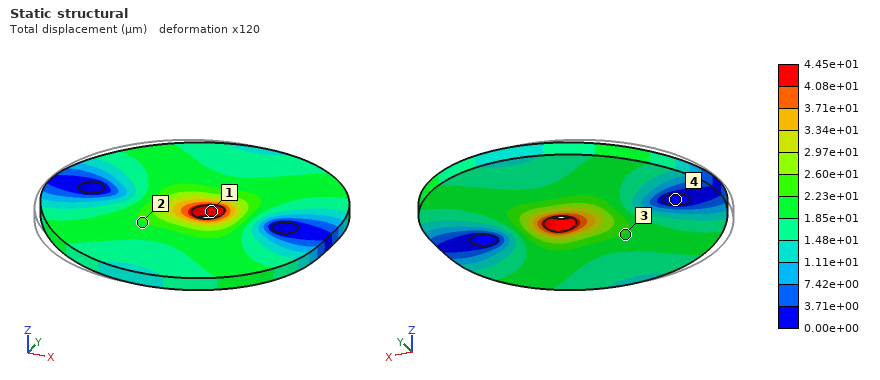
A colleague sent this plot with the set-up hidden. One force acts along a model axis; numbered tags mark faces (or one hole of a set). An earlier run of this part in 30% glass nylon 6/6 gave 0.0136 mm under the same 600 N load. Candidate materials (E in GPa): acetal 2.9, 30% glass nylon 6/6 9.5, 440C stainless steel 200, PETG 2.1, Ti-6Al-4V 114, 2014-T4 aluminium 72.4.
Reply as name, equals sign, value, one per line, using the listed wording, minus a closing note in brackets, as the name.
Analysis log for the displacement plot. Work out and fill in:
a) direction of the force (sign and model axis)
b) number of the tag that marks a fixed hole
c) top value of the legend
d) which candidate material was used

direction of the force = +X
number of the tag that marks a fixed hole = 4
top value of the legend = 4.45e+01 µm
which candidate material was used = acetal
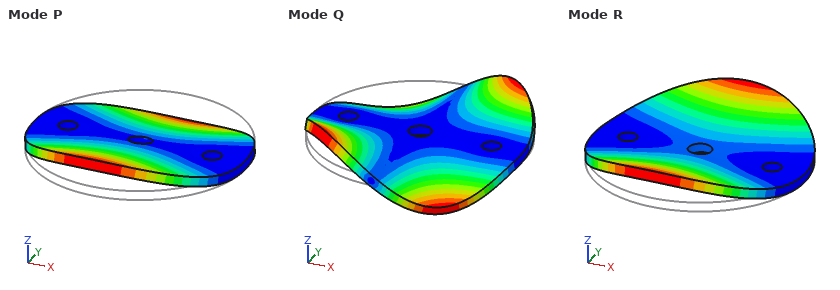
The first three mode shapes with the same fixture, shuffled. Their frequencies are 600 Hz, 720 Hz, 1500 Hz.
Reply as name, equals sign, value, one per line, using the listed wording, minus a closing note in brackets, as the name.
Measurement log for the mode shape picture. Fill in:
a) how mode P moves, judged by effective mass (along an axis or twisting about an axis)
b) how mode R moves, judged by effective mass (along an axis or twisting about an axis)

how mode P moves, judged by effective mass = twisting about X
how mode R moves, judged by effective mass = along Z
